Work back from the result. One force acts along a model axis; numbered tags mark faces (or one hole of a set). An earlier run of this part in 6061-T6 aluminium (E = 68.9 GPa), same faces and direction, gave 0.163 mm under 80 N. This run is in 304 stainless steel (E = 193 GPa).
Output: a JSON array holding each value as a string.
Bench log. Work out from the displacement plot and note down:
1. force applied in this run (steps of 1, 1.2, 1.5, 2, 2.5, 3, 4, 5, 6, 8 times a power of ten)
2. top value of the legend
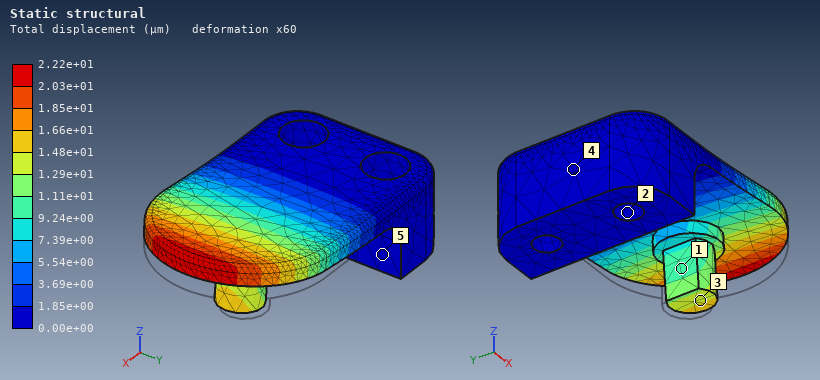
["30 N", "2.22e+01 µm"]
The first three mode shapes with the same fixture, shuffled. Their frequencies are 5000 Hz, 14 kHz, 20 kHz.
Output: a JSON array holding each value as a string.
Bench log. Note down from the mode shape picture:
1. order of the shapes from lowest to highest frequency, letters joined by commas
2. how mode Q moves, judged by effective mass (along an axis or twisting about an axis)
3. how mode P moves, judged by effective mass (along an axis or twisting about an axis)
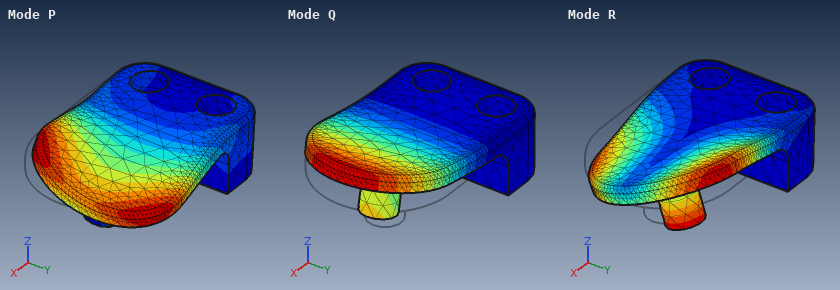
["Q, R, P", "along Z", "along Y"]
